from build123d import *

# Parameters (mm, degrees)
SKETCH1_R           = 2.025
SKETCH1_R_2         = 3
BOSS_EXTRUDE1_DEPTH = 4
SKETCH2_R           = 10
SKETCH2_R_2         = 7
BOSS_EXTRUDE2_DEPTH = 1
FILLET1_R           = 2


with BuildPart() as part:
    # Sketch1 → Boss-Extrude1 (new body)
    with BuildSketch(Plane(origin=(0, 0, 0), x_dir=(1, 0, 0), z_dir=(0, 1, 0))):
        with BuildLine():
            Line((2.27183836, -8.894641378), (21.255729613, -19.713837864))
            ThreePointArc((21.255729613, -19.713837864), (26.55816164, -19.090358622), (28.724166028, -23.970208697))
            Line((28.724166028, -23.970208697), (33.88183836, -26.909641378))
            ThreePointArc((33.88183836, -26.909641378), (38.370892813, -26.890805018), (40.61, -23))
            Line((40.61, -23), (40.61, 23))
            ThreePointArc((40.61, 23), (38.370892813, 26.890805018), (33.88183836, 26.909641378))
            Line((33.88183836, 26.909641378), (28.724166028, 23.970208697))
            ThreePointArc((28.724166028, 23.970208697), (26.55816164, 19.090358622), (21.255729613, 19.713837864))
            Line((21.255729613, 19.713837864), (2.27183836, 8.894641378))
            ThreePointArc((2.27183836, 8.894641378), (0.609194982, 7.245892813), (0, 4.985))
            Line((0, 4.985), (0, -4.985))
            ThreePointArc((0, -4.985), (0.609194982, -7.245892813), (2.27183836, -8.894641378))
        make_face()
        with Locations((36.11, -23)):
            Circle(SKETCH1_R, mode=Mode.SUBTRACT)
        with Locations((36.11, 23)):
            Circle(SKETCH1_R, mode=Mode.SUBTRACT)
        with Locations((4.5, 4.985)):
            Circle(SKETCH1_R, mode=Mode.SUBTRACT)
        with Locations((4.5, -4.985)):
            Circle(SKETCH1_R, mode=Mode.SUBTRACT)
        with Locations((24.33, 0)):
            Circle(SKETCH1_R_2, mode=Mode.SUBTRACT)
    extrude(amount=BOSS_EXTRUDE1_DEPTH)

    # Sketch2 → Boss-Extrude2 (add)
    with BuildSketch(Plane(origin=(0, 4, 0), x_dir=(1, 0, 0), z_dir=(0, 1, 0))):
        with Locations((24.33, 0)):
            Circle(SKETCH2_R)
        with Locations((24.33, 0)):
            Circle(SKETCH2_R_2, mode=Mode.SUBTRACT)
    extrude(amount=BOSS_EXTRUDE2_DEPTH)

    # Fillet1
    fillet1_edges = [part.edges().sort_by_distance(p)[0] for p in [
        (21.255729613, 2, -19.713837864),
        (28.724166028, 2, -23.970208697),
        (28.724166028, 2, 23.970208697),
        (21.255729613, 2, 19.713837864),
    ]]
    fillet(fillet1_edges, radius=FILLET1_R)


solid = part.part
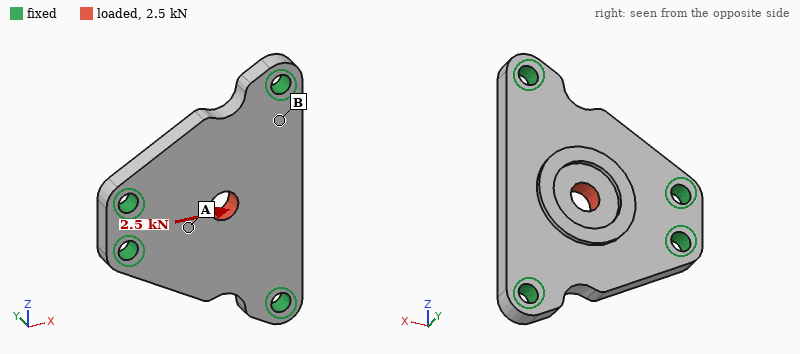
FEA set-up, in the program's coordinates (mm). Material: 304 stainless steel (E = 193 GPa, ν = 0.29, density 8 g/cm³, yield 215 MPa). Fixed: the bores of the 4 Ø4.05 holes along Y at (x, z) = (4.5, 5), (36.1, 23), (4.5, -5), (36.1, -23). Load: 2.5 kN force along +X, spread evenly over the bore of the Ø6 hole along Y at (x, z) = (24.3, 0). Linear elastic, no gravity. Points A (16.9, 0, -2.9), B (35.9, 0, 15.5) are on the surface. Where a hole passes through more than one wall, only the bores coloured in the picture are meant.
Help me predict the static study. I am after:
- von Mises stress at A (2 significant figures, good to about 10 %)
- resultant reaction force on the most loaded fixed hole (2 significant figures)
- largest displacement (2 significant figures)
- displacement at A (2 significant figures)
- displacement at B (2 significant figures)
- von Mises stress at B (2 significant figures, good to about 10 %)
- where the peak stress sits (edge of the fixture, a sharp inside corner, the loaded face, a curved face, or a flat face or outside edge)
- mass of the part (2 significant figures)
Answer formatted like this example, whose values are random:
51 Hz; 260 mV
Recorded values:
31 MPa; 930 N; 3.5 µm; 1.5 µm; 1.0 µm; 9.4 MPa; the loaded face; 46 g
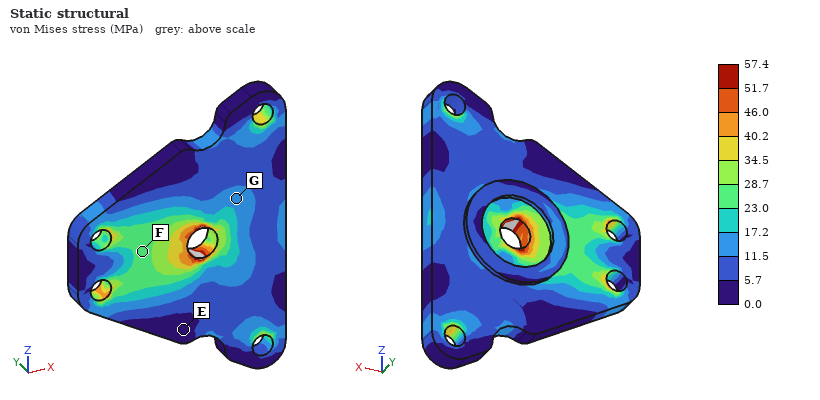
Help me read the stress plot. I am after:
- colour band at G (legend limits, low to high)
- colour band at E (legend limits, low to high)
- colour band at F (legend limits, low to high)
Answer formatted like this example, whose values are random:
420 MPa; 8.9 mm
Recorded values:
11.5 to 17.2 MPa; 0.0 to 5.7 MPa; 23.0 to 28.7 MPa
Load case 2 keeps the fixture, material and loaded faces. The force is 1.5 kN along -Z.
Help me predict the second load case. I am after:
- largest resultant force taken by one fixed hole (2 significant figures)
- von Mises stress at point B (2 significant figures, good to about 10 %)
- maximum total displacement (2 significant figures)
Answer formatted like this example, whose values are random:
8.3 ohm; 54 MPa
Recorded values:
540 N; 11 MPa; 1.8 µm
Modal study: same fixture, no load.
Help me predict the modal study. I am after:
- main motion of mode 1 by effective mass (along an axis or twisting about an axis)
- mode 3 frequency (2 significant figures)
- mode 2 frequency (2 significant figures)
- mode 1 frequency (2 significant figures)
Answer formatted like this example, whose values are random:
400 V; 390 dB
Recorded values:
along Y; 17 kHz; 17 kHz; 10 kHz
